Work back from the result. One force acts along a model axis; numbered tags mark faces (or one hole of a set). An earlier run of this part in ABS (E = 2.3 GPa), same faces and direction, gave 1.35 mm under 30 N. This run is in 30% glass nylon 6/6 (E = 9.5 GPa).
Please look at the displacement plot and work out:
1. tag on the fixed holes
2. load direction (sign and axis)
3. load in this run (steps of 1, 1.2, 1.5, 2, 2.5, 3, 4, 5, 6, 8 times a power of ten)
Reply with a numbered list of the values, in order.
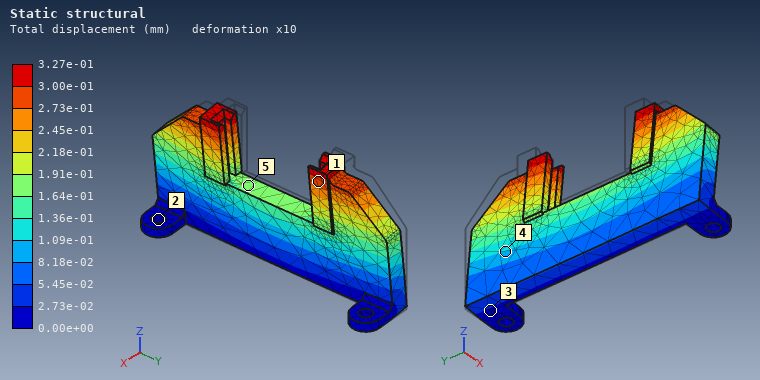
1. 2
2. +X
3. 30 N
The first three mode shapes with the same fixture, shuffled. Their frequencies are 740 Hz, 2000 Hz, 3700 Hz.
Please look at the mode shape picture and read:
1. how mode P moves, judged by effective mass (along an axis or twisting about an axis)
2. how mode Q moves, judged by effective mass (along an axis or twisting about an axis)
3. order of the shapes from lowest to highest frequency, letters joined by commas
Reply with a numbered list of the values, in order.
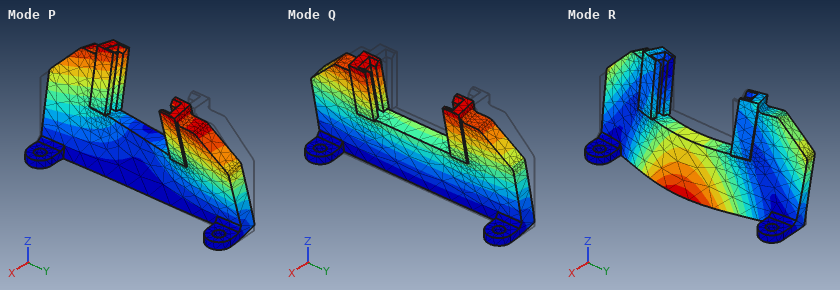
1. twisting about Z
2. along X
3. Q, P, R
